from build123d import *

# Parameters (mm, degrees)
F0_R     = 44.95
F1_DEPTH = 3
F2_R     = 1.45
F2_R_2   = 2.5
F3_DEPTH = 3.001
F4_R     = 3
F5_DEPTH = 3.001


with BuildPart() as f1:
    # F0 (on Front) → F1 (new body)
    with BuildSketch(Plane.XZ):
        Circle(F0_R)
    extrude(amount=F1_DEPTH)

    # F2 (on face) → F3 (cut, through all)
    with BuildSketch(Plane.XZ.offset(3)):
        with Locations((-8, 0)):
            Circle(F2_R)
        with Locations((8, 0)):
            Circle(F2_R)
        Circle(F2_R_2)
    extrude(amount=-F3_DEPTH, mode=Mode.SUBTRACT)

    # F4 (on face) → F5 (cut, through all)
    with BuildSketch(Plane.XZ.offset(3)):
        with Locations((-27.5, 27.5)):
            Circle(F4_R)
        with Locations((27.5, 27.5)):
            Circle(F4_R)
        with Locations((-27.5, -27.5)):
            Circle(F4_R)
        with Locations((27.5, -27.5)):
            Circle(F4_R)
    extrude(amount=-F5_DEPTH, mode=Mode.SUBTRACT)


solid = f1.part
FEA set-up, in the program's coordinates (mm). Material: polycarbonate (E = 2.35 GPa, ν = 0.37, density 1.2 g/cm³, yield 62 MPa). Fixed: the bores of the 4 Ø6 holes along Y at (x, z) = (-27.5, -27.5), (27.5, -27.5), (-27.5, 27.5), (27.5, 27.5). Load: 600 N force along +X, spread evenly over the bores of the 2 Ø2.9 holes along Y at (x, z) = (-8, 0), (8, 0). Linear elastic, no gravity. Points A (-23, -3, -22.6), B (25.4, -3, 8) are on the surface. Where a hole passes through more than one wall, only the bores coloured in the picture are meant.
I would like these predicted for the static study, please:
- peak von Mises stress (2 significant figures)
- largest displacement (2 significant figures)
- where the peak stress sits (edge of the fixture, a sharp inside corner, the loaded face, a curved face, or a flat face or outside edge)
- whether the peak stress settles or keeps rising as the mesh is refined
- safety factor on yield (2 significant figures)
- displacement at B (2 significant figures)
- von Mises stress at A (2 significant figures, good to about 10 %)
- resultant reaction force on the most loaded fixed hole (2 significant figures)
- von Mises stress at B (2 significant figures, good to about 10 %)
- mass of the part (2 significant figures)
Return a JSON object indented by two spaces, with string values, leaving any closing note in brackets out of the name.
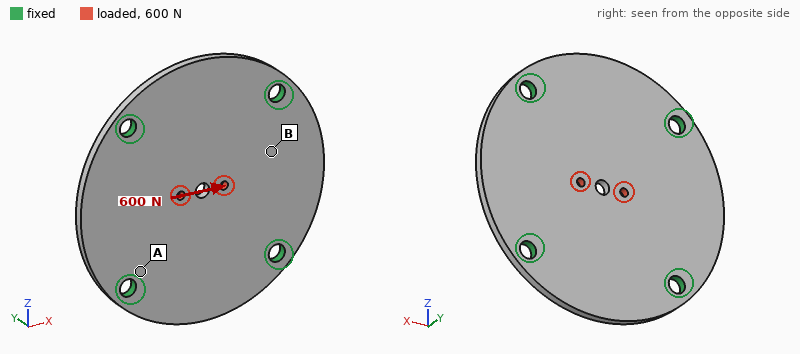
{
  "peak von Mises stress": "20 MPa",
  "largest displacement": "74 µm",
  "where the peak stress sits": "the loaded face",
  "whether the peak stress settles or keeps rising as the mesh is refined": "settles",
  "safety factor on yield": "3.1",
  "displacement at B": "34 µm",
  "von Mises stress at A": "4.0 MPa",
  "resultant reaction force on the most loaded fixed hole": "160 N",
  "von Mises stress at B": "1.8 MPa",
  "mass of the part": "22 g"
}
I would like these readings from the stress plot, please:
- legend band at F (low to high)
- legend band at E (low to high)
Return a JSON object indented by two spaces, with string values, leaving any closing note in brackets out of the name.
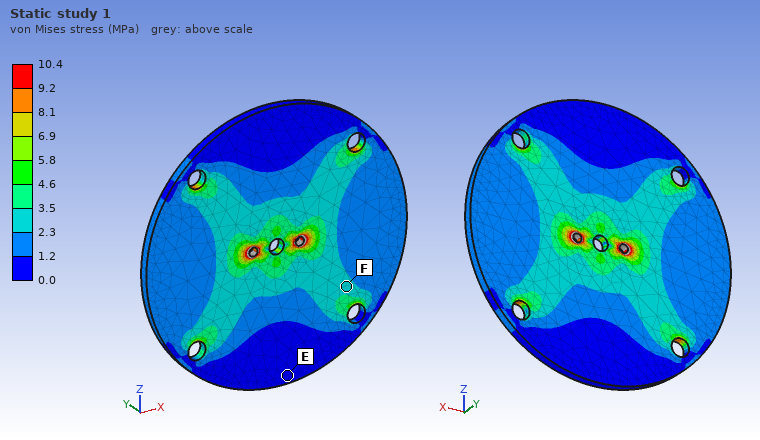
{
  "legend band at F": "2.3 to 3.5 MPa",
  "legend band at E": "0.0 to 1.2 MPa"
}
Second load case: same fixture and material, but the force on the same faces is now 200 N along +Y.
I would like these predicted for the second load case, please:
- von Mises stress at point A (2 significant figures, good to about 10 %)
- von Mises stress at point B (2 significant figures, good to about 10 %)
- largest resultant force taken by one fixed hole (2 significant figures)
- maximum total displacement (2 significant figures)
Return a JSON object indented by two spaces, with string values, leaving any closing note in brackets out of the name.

{
  "von Mises stress at point A": "14 MPa",
  "von Mises stress at point B": "6.9 MPa",
  "largest resultant force taken by one fixed hole": "50 N",
  "maximum total displacement": "1.2 mm"
}
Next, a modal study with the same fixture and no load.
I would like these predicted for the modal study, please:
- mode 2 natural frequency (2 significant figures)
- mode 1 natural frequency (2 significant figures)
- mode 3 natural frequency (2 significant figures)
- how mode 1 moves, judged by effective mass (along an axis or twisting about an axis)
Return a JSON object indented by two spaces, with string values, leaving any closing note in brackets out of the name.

{
  "mode 2 natural frequency": "1300 Hz",
  "mode 1 natural frequency": "1100 Hz",
  "mode 3 natural frequency": "1300 Hz",
  "how mode 1 moves, judged by effective mass": "along Y"
}
